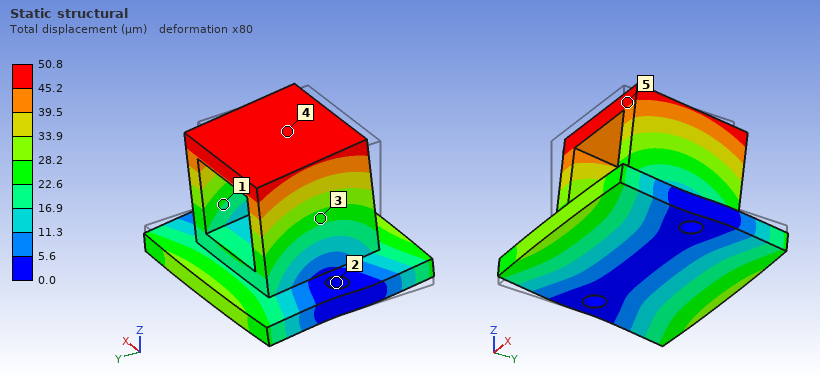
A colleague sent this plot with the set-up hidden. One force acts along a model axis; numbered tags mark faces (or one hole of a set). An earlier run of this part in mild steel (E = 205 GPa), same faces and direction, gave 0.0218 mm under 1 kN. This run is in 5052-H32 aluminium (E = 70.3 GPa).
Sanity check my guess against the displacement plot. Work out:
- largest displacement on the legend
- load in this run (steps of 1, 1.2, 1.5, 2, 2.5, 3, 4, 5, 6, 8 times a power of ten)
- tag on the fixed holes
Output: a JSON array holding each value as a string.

["50.8 µm", "800 N", "2"]
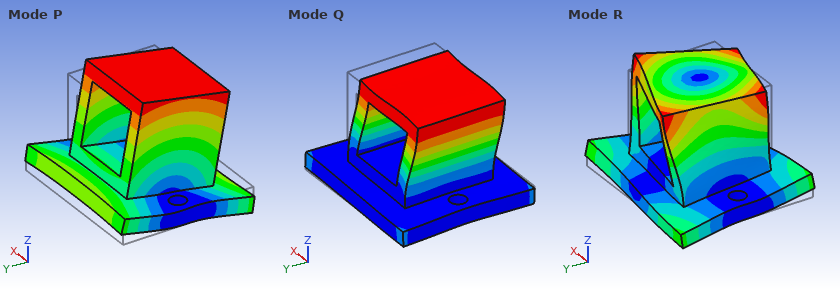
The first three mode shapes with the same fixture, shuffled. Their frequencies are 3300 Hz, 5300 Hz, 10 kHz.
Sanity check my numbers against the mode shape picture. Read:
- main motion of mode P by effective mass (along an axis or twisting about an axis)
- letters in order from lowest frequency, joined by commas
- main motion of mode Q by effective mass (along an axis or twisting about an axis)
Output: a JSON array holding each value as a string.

["along Y", "P, Q, R", "along X"]
